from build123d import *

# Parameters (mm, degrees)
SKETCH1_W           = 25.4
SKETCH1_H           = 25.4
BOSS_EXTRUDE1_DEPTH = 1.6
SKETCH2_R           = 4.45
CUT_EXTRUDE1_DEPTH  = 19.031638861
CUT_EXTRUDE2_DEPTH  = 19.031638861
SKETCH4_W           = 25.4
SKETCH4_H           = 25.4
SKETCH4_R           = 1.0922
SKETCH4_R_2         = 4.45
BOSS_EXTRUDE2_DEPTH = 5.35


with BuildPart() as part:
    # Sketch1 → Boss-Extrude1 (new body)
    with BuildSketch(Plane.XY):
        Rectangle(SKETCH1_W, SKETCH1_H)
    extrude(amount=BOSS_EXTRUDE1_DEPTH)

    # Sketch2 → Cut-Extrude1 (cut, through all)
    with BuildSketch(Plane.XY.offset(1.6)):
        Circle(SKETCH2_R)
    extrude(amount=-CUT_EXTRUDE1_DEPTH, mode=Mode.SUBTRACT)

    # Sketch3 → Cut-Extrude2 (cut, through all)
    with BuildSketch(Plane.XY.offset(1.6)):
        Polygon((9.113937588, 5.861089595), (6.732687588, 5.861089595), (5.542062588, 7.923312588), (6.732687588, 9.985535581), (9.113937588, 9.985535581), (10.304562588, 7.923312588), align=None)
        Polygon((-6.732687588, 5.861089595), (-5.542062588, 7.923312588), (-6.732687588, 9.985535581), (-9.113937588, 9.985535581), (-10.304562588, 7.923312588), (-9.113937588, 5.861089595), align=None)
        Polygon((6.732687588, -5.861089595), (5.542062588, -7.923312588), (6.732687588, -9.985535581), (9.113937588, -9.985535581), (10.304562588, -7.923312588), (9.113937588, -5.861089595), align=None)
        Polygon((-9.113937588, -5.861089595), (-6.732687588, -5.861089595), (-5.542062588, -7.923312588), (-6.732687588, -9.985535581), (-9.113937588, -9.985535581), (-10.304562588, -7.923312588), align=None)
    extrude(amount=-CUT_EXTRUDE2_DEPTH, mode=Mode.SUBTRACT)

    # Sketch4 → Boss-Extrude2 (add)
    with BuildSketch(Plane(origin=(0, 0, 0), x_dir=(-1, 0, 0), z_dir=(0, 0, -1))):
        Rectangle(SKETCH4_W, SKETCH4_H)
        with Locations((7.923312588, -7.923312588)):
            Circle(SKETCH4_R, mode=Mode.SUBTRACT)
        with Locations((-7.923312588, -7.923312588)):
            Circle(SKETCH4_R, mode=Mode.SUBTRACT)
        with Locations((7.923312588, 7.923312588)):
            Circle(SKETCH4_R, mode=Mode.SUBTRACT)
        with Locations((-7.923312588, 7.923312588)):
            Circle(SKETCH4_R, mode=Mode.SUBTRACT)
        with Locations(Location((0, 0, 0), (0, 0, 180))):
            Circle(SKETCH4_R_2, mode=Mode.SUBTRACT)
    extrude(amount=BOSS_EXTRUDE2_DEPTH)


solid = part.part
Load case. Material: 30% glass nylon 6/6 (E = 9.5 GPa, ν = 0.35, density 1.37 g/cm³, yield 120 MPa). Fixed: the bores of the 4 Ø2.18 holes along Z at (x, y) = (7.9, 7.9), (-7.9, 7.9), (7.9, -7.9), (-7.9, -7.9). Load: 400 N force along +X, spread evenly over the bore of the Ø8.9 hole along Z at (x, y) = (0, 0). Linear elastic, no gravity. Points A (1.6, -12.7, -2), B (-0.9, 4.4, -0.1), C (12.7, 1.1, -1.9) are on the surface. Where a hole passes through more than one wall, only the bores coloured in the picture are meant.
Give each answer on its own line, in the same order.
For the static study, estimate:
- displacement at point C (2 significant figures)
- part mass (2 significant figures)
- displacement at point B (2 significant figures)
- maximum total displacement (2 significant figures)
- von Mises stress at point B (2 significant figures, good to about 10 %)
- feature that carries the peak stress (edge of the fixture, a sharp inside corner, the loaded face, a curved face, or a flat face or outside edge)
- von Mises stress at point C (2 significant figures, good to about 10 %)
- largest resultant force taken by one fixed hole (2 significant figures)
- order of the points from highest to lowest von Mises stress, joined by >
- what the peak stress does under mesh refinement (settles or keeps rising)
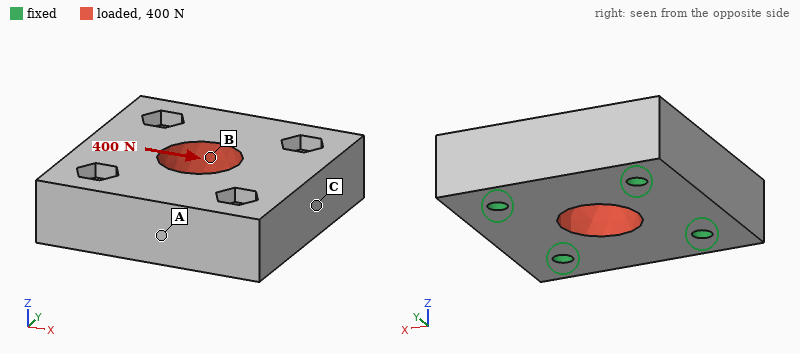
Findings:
2.1 µm
5.3 g
2.3 µm
3.4 µm
3.5 MPa
edge of the fixture
2.0 MPa
100 N
B > C > A
keeps rising
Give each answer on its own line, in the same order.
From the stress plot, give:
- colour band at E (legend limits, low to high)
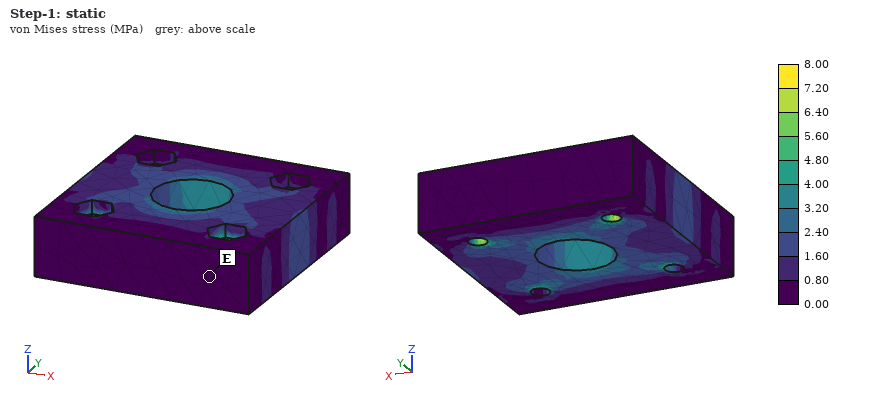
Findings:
0.00 to 0.80 MPa
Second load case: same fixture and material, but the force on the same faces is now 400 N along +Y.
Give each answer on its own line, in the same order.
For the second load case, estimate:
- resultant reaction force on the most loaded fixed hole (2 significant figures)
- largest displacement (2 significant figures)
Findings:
100 N
3.4 µm
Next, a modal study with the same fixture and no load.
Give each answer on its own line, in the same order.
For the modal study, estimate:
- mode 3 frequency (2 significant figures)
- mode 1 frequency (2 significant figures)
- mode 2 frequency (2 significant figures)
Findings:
34 kHz
31 kHz
32 kHz
